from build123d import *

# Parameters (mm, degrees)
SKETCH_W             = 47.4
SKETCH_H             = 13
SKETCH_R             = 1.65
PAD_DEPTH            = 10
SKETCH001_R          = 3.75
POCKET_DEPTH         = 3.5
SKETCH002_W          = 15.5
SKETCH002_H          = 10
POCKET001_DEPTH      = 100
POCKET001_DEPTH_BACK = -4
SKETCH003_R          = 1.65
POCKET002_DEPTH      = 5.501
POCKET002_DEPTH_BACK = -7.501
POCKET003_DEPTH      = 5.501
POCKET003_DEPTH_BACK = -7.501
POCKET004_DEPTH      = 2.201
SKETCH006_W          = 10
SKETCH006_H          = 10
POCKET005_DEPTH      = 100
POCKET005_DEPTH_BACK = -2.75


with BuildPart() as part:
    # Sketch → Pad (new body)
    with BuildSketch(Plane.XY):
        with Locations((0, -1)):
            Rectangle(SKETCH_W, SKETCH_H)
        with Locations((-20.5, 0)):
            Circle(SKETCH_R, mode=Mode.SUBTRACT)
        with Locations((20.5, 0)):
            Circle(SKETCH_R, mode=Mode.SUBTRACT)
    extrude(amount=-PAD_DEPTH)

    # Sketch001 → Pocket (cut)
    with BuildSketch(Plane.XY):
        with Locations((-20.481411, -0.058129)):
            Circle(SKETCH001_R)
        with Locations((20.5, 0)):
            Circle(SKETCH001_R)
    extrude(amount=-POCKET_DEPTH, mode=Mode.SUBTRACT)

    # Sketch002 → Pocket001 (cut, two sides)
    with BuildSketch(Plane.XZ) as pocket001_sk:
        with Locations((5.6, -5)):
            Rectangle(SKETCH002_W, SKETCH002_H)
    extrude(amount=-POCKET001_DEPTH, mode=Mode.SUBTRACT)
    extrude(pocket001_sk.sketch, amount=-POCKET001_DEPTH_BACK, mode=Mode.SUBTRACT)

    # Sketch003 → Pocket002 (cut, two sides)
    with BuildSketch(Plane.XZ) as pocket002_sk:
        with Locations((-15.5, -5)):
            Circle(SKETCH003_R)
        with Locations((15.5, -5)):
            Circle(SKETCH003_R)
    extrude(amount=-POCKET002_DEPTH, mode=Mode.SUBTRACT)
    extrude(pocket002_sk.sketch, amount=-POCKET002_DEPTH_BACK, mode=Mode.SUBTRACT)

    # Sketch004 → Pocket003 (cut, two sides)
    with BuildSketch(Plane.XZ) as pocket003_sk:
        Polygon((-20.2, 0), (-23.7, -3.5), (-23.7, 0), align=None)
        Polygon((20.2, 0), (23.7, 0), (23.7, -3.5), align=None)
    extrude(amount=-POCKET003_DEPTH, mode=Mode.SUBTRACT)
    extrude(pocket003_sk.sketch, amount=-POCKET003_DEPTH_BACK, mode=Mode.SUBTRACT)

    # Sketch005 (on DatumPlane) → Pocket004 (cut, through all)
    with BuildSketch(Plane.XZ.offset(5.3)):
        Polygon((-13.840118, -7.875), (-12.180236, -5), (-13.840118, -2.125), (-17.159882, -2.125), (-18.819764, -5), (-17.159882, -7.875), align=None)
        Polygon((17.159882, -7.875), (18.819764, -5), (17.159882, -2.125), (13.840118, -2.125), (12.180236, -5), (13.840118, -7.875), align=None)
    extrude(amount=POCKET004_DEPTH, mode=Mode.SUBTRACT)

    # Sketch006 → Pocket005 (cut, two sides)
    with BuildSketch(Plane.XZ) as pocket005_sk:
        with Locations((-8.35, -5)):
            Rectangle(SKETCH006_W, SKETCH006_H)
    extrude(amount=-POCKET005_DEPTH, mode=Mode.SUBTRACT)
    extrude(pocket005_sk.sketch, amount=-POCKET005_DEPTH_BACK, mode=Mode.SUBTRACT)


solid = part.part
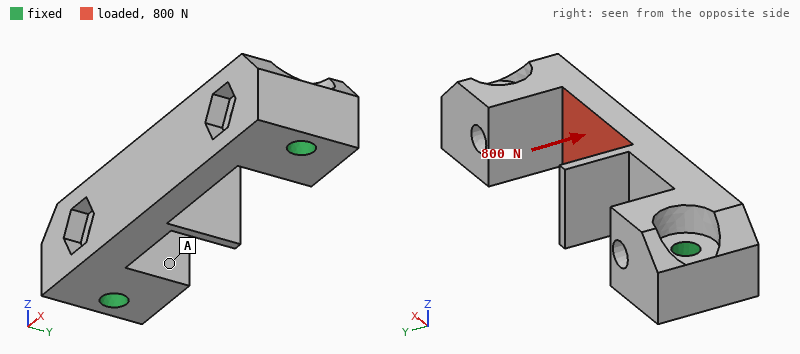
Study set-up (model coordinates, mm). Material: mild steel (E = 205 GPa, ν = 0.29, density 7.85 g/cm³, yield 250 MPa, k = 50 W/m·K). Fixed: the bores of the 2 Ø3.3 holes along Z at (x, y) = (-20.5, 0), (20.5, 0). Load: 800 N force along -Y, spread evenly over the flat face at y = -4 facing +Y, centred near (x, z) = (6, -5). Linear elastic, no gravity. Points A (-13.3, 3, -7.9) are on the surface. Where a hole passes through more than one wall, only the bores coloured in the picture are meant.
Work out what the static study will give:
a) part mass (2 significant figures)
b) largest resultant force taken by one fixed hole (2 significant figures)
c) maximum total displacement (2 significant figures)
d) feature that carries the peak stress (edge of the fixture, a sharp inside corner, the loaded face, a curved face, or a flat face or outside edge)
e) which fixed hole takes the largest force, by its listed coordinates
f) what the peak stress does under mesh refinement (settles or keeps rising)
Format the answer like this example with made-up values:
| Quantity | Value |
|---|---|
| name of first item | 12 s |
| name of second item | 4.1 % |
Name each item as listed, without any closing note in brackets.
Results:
| Quantity | Value |
|---|---|
| part mass | 24 g |
| largest resultant force taken by one fixed hole | 700 N |
| maximum total displacement | 15 µm |
| feature that carries the peak stress | a sharp inside corner |
| which fixed hole takes the largest force, by its listed coordinates | (20.5, 0) |
| what the peak stress does under mesh refinement | keeps rising |
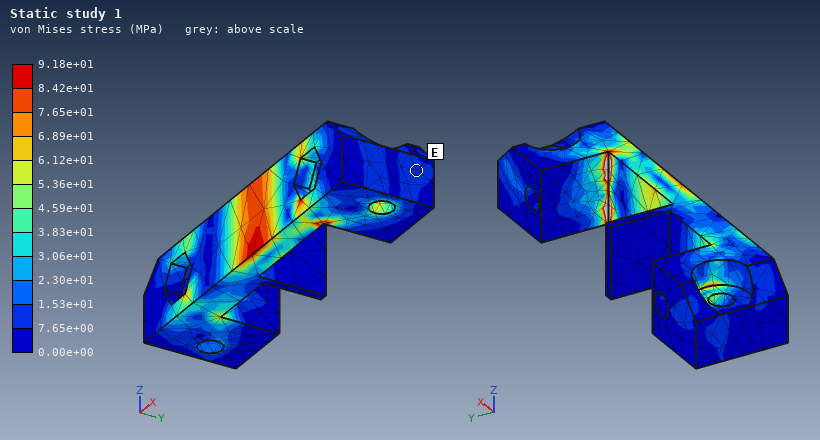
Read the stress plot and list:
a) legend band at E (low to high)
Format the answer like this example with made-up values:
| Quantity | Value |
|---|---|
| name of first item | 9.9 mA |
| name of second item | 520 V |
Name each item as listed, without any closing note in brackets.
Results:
| Quantity | Value |
|---|---|
| legend band at E | 7.65e+00 to 1.53e+01 MPa |
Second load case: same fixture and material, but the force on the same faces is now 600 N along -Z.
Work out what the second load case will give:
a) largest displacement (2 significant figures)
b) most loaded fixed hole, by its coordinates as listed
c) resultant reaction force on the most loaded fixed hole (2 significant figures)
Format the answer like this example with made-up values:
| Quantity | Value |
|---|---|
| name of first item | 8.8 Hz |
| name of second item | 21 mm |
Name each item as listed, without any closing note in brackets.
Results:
| Quantity | Value |
|---|---|
| largest displacement | 6.5 µm |
| most loaded fixed hole, by its coordinates as listed | (20.5, 0) |
| resultant reaction force on the most loaded fixed hole | 400 N |
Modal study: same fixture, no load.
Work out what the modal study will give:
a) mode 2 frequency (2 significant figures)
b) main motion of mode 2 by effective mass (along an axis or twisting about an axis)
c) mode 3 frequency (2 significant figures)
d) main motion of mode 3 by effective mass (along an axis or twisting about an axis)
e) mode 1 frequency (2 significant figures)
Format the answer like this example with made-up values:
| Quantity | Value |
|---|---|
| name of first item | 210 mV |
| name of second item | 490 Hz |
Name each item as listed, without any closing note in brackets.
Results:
| Quantity | Value |
|---|---|
| mode 2 frequency | 15 kHz |
| main motion of mode 2 by effective mass | along Y |
| mode 3 frequency | 18 kHz |
| main motion of mode 3 by effective mass | along Z |
| mode 1 frequency | 13 kHz |
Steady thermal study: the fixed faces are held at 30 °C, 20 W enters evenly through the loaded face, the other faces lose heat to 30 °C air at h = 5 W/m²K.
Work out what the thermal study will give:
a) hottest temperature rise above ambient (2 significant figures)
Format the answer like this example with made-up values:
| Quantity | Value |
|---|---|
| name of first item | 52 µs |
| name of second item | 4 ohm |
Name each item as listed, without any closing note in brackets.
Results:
| Quantity | Value |
|---|---|
| hottest temperature rise above ambient | 84 K |
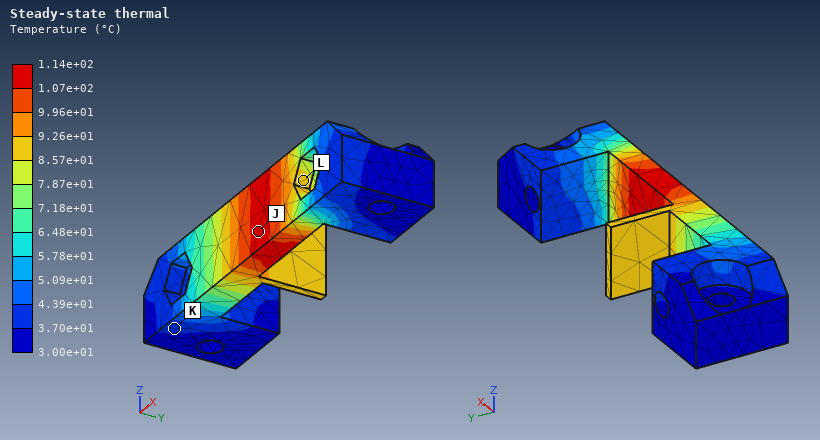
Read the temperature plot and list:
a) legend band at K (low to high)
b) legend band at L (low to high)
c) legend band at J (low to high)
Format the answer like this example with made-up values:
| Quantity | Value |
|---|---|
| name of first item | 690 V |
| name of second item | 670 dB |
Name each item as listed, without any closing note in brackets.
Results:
| Quantity | Value |
|---|---|
| legend band at K | 3.70e+01 to 4.39e+01 °C |
| legend band at L | 8.57e+01 to 9.26e+01 °C |
| legend band at J | 1.07e+02 to 1.14e+02 °C |
